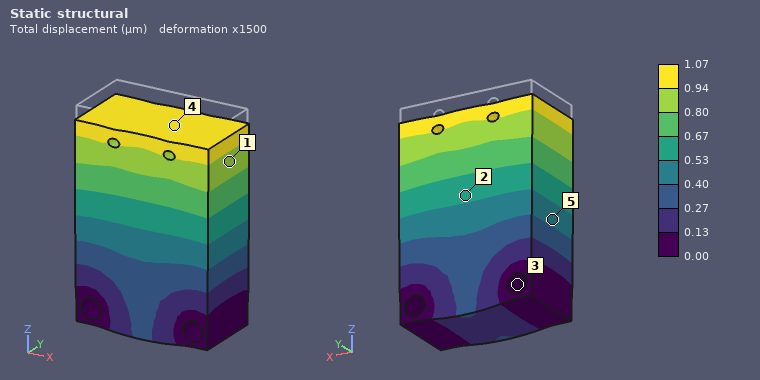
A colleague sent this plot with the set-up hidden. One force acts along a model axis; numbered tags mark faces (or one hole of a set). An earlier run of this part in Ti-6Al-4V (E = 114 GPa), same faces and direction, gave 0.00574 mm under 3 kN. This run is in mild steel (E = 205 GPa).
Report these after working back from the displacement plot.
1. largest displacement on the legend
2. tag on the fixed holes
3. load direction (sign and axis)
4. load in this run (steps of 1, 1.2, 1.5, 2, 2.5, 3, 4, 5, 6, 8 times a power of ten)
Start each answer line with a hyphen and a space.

- 1.07 µm
- 3
- -Z
- 1 kN
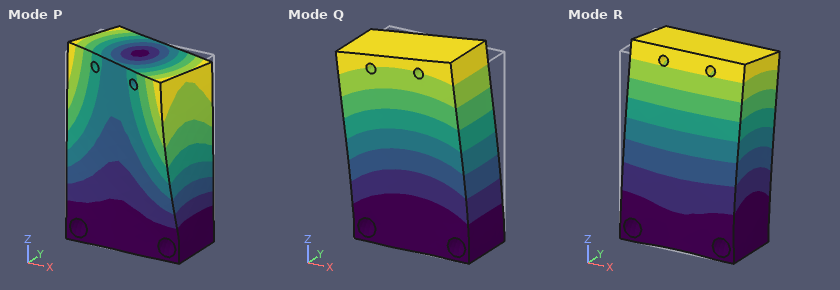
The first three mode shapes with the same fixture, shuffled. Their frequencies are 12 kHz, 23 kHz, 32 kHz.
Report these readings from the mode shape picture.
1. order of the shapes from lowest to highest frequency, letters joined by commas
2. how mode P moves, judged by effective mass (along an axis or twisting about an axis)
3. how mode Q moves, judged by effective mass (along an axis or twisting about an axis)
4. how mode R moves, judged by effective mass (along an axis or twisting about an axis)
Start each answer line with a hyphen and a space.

- R, Q, P
- twisting about Z
- along X
- along Y
